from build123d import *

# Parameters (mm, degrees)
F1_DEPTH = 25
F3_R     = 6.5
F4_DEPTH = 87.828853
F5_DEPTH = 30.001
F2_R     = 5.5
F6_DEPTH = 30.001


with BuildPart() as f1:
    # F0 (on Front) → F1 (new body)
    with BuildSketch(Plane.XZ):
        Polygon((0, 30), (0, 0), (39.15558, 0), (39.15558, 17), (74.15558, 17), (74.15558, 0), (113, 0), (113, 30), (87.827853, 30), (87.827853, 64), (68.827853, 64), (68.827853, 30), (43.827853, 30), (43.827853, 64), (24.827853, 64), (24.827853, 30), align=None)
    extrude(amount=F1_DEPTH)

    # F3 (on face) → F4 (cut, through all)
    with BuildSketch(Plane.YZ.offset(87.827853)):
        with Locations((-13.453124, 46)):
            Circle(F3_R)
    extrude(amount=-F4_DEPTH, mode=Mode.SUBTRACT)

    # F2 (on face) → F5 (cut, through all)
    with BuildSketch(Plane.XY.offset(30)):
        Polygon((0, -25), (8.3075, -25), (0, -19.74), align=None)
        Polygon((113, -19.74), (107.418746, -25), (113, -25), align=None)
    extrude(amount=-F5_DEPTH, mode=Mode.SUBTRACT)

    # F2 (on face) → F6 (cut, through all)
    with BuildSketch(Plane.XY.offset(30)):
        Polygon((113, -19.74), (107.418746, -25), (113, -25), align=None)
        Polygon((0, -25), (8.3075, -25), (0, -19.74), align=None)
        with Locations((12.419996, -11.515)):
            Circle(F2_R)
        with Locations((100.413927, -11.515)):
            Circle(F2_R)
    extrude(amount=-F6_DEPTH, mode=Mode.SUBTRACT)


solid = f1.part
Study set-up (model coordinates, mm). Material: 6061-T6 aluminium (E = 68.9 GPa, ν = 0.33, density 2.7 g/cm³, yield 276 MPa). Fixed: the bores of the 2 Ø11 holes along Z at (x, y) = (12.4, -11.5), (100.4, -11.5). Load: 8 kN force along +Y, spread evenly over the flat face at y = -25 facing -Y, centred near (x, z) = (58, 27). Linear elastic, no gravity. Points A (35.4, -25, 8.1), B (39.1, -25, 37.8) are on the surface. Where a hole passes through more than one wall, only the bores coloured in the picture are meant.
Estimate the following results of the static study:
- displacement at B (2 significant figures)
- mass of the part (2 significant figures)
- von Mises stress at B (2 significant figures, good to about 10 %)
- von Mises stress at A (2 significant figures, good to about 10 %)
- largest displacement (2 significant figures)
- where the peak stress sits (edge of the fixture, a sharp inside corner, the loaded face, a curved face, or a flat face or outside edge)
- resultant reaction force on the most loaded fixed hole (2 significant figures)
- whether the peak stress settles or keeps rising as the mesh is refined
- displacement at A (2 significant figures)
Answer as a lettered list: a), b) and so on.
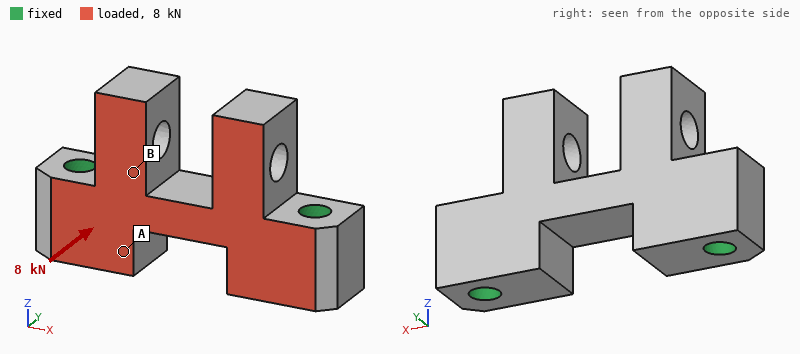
a) 22 µm
b) 240 g
c) 15 MPa
d) 6.1 MPa
e) 45 µm
f) edge of the fixture
g) 4.1 kN
h) keeps rising
i) 7.0 µm
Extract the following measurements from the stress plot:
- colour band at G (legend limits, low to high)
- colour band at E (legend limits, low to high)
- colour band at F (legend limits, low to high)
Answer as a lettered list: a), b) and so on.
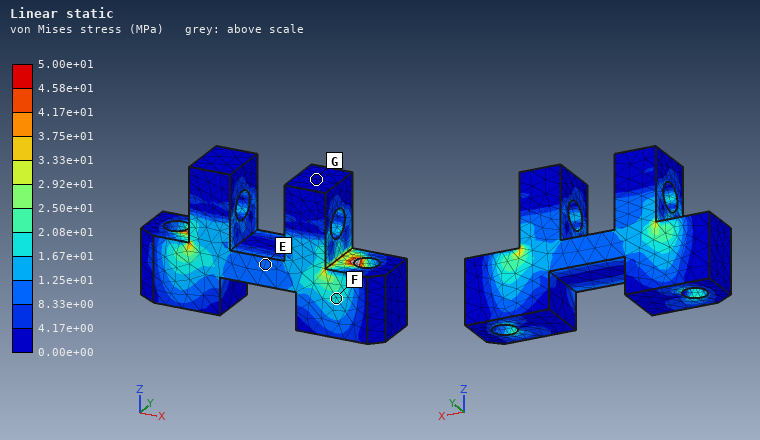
a) 0.00e+00 to 4.17e+00 MPa
b) 8.33e+00 to 1.25e+01 MPa
c) 1.67e+01 to 2.08e+01 MPa
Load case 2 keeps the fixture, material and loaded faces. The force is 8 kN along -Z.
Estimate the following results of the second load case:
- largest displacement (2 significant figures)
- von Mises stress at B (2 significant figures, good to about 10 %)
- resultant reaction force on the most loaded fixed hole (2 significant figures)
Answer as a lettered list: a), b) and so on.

a) 32 µm
b) 12 MPa
c) 4.2 kN
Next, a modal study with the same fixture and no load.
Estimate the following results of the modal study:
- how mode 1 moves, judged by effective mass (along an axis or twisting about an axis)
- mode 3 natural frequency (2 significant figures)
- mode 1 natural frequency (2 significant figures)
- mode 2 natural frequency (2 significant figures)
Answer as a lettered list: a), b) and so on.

a) along Y
b) 6600 Hz
c) 5700 Hz
d) 6500 Hz
